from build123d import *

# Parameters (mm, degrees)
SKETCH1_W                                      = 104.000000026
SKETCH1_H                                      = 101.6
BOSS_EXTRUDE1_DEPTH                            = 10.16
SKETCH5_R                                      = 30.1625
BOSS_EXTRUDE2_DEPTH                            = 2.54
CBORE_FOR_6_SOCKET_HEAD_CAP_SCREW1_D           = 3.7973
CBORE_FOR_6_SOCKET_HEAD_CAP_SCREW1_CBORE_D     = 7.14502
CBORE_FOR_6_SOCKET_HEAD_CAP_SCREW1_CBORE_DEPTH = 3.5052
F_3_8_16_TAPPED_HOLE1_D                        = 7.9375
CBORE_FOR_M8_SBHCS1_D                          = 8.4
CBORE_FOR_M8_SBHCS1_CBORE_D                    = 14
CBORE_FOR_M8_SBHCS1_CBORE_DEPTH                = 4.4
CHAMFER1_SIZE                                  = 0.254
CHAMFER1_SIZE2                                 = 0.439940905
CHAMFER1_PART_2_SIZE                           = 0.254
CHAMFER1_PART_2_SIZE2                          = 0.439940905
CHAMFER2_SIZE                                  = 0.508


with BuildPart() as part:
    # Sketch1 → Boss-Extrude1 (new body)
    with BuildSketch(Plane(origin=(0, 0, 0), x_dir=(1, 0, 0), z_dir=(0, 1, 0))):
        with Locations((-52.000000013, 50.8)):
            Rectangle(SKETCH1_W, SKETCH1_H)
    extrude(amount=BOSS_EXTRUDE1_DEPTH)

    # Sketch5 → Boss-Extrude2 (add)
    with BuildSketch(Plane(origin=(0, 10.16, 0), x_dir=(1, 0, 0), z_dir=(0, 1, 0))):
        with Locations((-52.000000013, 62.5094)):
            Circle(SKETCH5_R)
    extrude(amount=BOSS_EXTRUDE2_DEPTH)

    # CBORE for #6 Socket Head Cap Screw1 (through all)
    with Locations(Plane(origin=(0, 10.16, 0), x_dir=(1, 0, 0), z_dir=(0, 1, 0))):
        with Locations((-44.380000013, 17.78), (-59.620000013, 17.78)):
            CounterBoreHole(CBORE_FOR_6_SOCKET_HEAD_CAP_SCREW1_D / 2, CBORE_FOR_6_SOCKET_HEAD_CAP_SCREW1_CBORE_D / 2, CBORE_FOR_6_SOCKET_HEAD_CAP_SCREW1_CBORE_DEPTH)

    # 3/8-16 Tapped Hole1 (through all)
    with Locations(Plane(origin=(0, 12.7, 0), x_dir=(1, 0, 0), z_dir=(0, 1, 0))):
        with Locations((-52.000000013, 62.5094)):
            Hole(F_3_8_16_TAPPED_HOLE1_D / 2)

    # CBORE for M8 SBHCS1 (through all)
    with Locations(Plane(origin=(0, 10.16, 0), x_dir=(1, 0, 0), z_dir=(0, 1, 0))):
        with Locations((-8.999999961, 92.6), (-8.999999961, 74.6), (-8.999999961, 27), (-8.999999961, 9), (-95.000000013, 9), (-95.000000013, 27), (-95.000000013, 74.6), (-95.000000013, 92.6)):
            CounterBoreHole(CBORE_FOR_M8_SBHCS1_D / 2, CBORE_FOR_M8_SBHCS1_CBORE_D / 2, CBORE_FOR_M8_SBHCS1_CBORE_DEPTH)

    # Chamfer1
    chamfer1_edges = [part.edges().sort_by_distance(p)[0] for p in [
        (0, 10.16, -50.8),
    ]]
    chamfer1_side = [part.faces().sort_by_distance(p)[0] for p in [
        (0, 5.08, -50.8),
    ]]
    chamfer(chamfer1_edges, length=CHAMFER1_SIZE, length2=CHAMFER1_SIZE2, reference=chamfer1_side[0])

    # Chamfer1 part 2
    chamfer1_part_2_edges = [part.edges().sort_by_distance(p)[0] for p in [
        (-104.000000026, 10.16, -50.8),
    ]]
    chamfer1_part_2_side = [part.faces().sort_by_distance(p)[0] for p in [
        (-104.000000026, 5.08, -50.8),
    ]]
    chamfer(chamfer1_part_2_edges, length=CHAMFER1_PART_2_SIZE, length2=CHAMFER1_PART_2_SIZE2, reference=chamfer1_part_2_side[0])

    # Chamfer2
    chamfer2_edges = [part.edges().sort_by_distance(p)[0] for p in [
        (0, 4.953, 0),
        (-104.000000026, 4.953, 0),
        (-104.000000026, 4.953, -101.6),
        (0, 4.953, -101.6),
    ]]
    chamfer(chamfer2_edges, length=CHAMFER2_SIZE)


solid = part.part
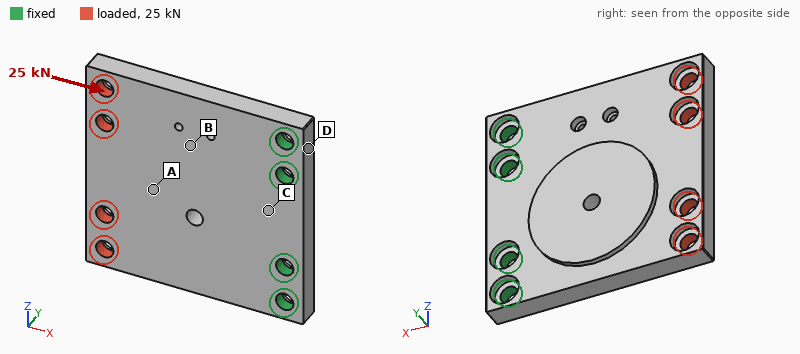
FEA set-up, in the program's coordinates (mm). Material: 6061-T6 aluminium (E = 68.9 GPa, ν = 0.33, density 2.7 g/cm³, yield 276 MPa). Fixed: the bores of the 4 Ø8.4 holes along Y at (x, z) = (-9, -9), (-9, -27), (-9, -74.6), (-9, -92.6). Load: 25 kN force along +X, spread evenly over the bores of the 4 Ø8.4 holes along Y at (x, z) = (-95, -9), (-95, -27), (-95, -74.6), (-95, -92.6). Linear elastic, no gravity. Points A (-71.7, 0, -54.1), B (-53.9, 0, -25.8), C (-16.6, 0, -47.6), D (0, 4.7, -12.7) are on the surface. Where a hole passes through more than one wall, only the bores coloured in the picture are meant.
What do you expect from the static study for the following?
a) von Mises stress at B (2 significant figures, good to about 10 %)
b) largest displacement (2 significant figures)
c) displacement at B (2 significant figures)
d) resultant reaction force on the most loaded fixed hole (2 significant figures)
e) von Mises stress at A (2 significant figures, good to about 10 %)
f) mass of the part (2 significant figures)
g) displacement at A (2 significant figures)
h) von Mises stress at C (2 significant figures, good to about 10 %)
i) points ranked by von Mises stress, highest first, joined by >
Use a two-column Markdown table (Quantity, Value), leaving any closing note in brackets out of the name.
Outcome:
| Quantity | Value |
|---|---|
| von Mises stress at B | 55 MPa |
| largest displacement | 0.34 mm |
| displacement at B | 0.076 mm |
| resultant reaction force on the most loaded fixed hole | 7.0 kN |
| von Mises stress at A | 37 MPa |
| mass of the part | 290 g |
| displacement at A | 0.15 mm |
| von Mises stress at C | 23 MPa |
| points ranked by von Mises stress, highest first, joined by > | B > A > C > D |
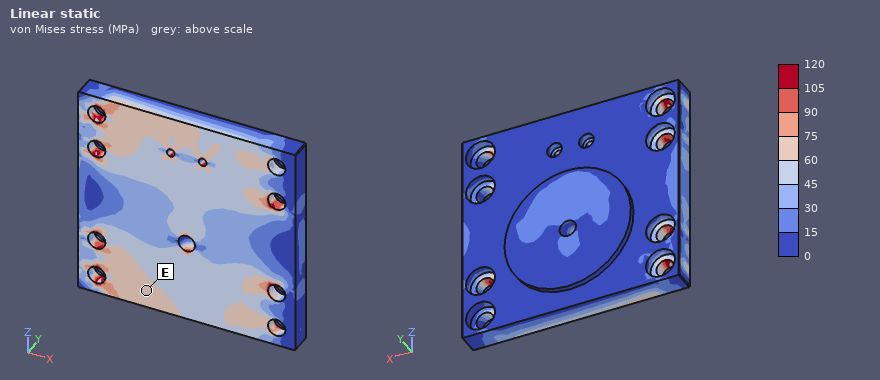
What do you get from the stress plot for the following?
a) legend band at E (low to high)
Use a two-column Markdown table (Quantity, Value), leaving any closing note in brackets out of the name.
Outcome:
| Quantity | Value |
|---|---|
| legend band at E | 60 to 75 MPa |
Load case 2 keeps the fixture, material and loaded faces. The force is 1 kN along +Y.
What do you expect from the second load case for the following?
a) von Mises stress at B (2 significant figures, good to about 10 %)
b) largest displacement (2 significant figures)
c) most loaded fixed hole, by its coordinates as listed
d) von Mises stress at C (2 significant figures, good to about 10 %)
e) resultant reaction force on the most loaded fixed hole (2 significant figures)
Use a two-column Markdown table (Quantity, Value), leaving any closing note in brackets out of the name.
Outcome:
| Quantity | Value |
|---|---|
| von Mises stress at B | 18 MPa |
| largest displacement | 0.49 mm |
| most loaded fixed hole, by its coordinates as listed | (-9, -27) |
| von Mises stress at C | 28 MPa |
| resultant reaction force on the most loaded fixed hole | 520 N |
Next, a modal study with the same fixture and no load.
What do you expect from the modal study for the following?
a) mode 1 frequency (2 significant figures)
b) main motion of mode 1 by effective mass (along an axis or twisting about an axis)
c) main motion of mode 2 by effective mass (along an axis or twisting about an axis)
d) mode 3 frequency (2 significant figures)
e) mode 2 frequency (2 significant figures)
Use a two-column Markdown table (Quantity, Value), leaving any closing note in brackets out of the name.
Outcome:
| Quantity | Value |
|---|---|
| mode 1 frequency | 830 Hz |
| main motion of mode 1 by effective mass | along Y |
| main motion of mode 2 by effective mass | twisting about X |
| mode 3 frequency | 5400 Hz |
| mode 2 frequency | 2300 Hz |
